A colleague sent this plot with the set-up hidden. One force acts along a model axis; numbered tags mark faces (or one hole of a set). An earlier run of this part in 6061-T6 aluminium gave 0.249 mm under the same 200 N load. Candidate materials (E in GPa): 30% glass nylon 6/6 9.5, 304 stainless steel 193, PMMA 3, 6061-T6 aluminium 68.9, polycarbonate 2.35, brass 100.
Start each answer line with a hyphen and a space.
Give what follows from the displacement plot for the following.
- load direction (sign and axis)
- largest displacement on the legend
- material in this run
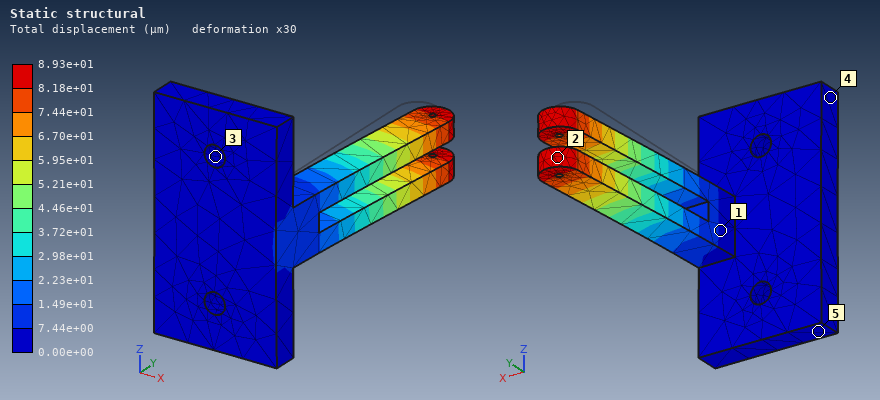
- +X
- 8.93e+01 µm
- 304 stainless steel
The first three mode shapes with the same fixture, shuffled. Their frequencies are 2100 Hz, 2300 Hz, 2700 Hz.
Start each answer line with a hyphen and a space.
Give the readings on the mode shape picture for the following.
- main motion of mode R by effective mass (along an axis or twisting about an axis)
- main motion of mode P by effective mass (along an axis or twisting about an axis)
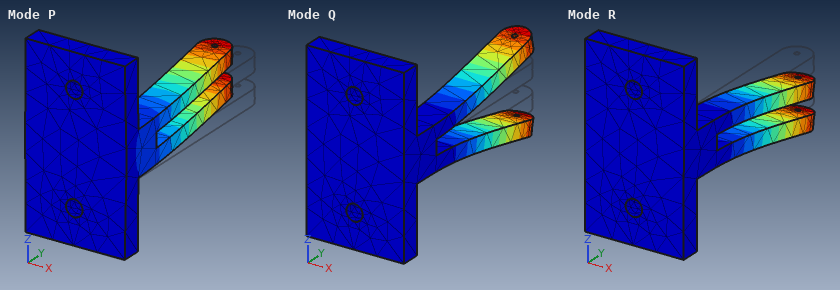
- along Z
- along X
